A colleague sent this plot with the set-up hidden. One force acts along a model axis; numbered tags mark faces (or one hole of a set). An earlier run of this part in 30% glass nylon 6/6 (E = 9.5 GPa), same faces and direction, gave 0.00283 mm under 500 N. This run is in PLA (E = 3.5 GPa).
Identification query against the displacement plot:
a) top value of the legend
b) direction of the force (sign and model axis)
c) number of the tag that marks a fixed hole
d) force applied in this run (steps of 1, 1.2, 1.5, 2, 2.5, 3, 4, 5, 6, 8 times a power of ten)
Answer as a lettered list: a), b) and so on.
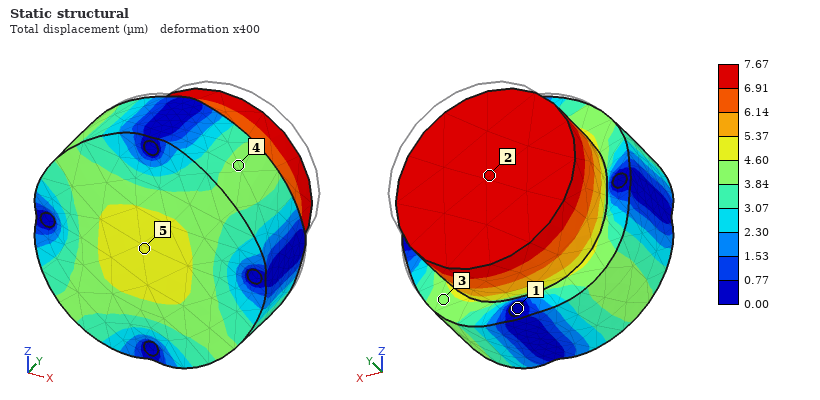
a) 7.67 µm
b) -Y
c) 1
d) 500 N
